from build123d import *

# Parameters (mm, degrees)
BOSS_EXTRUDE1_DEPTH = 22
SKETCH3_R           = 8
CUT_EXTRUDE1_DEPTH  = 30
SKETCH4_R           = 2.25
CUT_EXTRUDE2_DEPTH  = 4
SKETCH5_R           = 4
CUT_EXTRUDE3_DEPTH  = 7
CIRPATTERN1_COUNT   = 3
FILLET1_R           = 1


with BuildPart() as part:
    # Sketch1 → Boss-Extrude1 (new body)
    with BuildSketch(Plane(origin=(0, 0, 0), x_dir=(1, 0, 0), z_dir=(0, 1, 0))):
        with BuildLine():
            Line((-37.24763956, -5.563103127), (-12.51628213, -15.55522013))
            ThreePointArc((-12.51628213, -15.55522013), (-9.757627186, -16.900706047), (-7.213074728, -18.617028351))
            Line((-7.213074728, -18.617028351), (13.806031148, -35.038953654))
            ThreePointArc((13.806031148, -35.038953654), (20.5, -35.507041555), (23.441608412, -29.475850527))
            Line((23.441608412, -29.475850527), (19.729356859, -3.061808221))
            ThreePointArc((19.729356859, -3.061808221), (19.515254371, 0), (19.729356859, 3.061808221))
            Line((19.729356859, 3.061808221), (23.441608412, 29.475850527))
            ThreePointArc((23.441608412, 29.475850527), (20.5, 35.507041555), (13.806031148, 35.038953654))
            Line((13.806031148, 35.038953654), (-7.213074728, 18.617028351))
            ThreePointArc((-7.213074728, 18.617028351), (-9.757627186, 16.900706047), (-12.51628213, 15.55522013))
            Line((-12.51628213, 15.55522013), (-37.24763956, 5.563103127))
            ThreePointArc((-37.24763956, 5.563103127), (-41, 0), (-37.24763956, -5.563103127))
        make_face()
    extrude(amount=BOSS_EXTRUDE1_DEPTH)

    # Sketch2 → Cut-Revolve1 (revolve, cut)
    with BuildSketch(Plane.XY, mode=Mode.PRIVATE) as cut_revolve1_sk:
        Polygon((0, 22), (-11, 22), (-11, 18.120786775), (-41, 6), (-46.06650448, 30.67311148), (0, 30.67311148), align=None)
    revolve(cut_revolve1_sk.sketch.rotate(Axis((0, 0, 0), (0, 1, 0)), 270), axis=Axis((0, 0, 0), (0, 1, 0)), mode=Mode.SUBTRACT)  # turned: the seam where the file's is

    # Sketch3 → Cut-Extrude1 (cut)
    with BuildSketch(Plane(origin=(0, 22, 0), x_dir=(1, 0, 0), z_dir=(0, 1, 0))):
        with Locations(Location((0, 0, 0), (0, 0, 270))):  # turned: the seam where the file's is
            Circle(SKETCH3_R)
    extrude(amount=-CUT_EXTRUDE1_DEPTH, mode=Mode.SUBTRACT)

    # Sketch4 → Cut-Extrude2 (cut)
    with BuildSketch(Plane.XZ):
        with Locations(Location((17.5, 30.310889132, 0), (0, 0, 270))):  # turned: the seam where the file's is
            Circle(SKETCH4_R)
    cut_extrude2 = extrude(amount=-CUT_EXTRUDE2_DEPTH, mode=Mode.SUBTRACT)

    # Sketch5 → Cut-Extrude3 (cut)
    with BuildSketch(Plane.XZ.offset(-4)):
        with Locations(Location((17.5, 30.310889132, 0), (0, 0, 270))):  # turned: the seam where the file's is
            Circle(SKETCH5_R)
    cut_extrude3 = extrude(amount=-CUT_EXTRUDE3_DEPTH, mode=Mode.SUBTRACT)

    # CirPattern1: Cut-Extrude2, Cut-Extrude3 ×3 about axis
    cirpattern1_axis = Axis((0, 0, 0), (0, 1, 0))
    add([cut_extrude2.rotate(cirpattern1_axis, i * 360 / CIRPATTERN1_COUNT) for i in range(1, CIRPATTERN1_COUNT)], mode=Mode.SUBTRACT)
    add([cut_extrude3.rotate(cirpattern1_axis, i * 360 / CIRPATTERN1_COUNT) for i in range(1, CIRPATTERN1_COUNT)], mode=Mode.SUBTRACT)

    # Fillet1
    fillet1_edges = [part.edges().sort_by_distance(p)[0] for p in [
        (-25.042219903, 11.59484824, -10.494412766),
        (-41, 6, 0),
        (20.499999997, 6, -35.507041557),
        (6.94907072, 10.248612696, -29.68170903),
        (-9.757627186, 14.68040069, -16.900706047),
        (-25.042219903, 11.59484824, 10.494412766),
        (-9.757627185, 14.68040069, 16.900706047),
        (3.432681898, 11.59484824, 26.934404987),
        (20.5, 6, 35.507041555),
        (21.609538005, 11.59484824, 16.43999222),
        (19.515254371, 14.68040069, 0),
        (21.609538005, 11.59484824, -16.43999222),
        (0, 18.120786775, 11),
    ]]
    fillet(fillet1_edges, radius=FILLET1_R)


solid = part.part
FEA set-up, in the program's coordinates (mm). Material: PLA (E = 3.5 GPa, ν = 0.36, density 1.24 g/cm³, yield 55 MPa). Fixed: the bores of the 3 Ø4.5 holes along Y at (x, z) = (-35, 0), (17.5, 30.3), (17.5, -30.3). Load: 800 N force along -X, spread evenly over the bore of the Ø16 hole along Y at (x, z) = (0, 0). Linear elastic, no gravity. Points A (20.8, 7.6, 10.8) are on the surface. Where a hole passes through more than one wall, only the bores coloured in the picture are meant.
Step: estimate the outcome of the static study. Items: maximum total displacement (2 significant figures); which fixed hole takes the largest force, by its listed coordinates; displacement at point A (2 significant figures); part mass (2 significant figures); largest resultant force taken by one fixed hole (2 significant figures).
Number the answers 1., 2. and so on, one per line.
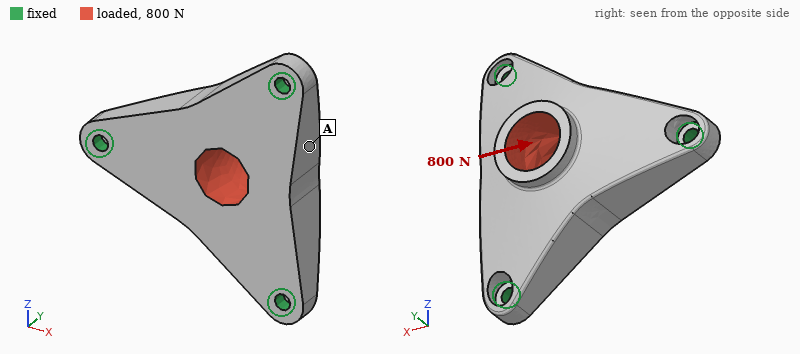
1. 54 µm
2. (-35, 0)
3. 32 µm
4. 37 g
5. 450 N
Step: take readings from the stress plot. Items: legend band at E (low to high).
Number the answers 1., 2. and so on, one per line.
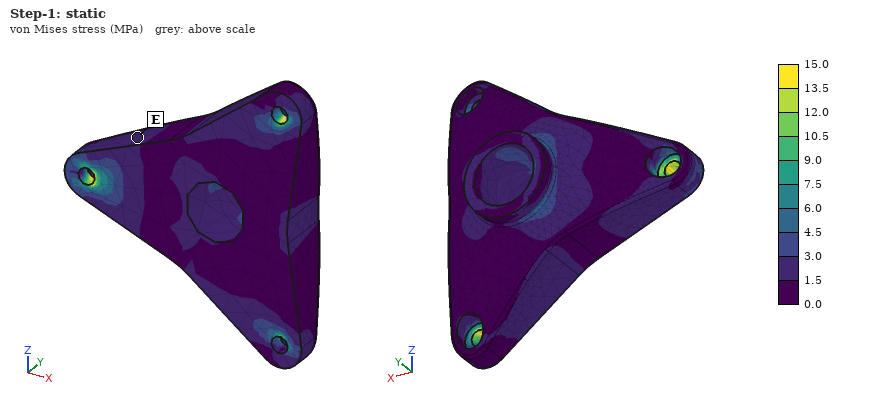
1. 1.5 to 3.0 MPa
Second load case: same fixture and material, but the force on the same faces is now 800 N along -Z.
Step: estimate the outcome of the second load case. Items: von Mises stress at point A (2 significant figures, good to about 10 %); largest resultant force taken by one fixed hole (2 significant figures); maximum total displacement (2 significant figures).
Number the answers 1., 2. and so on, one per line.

1. 2.0 MPa
2. 390 N
3. 50 µm
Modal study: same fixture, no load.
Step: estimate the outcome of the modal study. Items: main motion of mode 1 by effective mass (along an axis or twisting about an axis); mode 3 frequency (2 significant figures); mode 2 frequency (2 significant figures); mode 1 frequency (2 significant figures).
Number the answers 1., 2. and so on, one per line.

1. along Y
2. 4900 Hz
3. 4900 Hz
4. 3300 Hz
